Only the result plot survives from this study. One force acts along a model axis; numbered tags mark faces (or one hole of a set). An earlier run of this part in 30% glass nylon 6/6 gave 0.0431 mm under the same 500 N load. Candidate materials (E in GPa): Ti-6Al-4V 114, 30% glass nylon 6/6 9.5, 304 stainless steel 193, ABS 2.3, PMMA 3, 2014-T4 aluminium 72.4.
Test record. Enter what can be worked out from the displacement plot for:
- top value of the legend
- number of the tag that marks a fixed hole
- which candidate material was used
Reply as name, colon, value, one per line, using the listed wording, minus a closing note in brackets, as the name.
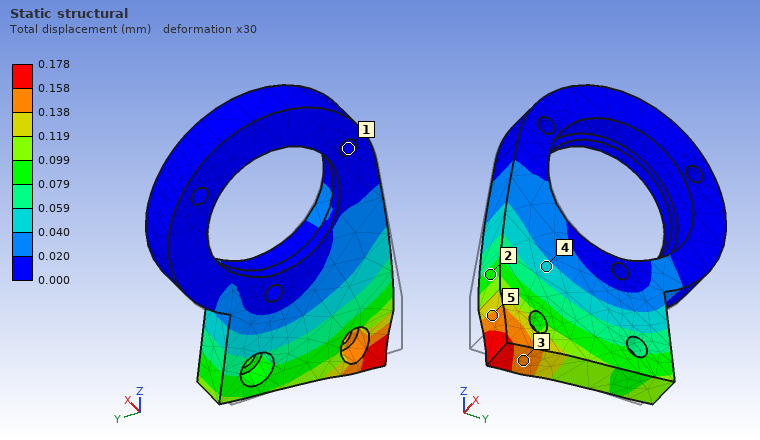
top value of the legend: 0.178 mm
number of the tag that marks a fixed hole: 1
which candidate material was used: ABS
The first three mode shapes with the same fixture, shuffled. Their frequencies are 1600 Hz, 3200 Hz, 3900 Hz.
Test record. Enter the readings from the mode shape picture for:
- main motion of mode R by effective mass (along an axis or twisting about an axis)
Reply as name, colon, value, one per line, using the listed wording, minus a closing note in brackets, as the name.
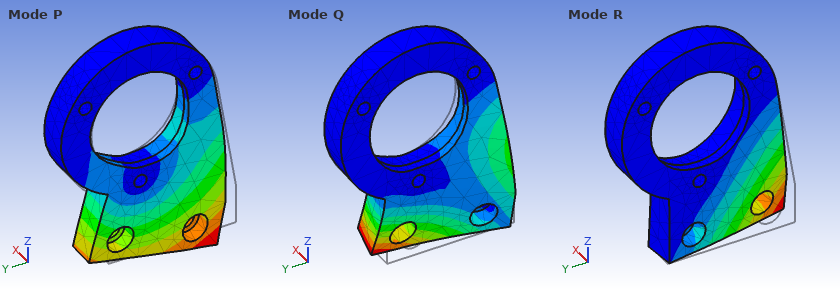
main motion of mode R by effective mass: along X
